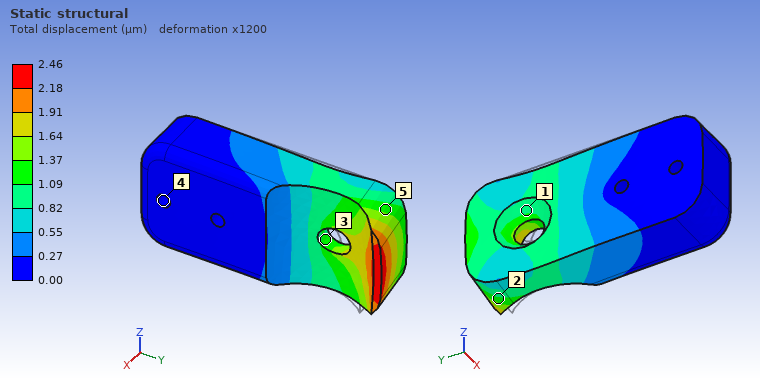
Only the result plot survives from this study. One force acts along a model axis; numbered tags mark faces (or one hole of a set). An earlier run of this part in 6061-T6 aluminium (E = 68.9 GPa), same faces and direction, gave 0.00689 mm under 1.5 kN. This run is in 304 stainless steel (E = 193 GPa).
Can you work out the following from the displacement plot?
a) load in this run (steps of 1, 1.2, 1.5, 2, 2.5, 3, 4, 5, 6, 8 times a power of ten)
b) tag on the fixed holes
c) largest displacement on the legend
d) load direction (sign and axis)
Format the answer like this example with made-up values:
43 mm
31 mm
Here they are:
1.5 kN
4
2.46 µm
+Y
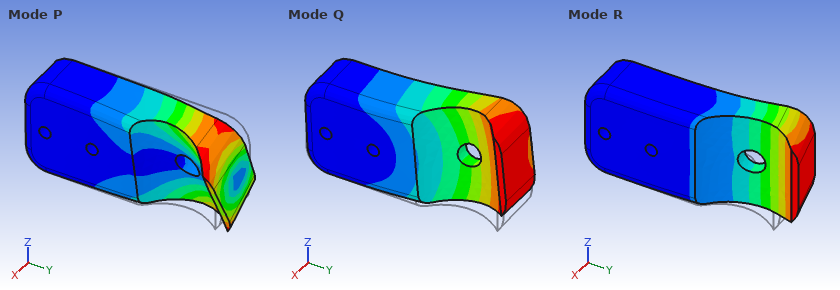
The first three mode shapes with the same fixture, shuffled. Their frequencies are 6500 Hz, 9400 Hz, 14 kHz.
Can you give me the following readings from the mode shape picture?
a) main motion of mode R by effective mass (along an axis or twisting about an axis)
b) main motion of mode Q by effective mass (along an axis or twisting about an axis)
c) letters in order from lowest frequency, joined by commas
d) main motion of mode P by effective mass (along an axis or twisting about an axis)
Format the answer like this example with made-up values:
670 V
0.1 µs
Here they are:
along X
along Z
R, Q, P
twisting about Y
